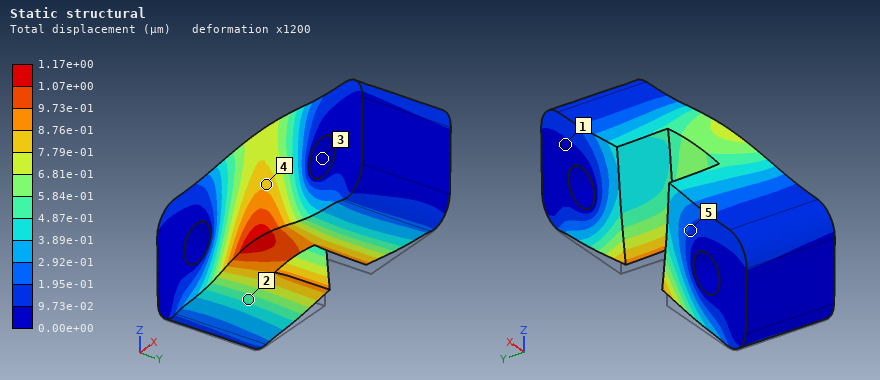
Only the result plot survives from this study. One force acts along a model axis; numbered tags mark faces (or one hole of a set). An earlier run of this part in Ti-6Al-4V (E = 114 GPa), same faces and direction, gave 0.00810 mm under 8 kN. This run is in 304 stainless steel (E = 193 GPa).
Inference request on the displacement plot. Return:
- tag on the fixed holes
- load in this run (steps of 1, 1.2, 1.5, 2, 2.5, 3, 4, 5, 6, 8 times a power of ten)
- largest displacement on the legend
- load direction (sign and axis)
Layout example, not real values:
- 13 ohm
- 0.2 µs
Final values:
- 3
- 2 kN
- 1.17e+00 µm
- +Z
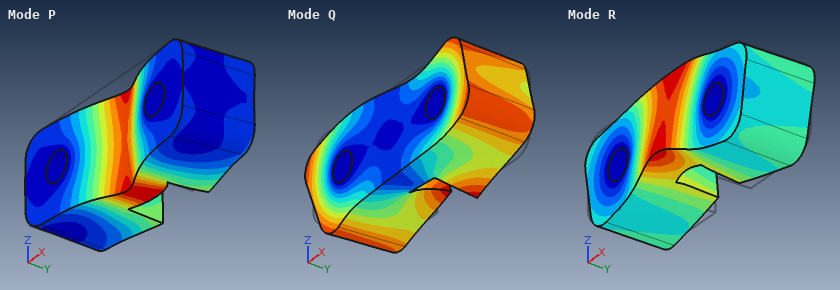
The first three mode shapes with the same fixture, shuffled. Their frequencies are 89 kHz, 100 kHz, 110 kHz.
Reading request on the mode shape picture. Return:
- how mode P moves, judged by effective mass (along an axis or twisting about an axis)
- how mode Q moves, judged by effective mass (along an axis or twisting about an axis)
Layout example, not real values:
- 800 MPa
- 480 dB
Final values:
- along Y
- twisting about Y
